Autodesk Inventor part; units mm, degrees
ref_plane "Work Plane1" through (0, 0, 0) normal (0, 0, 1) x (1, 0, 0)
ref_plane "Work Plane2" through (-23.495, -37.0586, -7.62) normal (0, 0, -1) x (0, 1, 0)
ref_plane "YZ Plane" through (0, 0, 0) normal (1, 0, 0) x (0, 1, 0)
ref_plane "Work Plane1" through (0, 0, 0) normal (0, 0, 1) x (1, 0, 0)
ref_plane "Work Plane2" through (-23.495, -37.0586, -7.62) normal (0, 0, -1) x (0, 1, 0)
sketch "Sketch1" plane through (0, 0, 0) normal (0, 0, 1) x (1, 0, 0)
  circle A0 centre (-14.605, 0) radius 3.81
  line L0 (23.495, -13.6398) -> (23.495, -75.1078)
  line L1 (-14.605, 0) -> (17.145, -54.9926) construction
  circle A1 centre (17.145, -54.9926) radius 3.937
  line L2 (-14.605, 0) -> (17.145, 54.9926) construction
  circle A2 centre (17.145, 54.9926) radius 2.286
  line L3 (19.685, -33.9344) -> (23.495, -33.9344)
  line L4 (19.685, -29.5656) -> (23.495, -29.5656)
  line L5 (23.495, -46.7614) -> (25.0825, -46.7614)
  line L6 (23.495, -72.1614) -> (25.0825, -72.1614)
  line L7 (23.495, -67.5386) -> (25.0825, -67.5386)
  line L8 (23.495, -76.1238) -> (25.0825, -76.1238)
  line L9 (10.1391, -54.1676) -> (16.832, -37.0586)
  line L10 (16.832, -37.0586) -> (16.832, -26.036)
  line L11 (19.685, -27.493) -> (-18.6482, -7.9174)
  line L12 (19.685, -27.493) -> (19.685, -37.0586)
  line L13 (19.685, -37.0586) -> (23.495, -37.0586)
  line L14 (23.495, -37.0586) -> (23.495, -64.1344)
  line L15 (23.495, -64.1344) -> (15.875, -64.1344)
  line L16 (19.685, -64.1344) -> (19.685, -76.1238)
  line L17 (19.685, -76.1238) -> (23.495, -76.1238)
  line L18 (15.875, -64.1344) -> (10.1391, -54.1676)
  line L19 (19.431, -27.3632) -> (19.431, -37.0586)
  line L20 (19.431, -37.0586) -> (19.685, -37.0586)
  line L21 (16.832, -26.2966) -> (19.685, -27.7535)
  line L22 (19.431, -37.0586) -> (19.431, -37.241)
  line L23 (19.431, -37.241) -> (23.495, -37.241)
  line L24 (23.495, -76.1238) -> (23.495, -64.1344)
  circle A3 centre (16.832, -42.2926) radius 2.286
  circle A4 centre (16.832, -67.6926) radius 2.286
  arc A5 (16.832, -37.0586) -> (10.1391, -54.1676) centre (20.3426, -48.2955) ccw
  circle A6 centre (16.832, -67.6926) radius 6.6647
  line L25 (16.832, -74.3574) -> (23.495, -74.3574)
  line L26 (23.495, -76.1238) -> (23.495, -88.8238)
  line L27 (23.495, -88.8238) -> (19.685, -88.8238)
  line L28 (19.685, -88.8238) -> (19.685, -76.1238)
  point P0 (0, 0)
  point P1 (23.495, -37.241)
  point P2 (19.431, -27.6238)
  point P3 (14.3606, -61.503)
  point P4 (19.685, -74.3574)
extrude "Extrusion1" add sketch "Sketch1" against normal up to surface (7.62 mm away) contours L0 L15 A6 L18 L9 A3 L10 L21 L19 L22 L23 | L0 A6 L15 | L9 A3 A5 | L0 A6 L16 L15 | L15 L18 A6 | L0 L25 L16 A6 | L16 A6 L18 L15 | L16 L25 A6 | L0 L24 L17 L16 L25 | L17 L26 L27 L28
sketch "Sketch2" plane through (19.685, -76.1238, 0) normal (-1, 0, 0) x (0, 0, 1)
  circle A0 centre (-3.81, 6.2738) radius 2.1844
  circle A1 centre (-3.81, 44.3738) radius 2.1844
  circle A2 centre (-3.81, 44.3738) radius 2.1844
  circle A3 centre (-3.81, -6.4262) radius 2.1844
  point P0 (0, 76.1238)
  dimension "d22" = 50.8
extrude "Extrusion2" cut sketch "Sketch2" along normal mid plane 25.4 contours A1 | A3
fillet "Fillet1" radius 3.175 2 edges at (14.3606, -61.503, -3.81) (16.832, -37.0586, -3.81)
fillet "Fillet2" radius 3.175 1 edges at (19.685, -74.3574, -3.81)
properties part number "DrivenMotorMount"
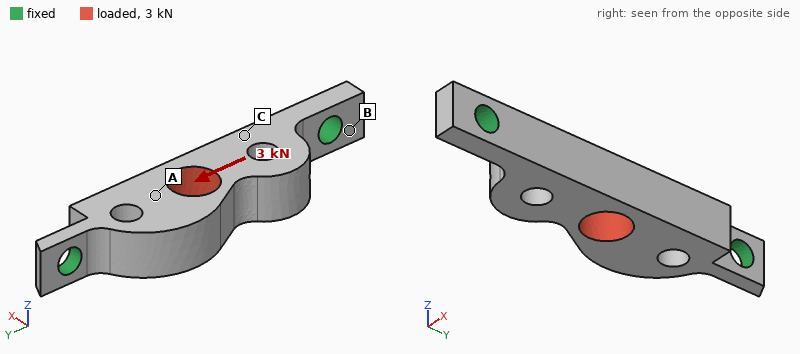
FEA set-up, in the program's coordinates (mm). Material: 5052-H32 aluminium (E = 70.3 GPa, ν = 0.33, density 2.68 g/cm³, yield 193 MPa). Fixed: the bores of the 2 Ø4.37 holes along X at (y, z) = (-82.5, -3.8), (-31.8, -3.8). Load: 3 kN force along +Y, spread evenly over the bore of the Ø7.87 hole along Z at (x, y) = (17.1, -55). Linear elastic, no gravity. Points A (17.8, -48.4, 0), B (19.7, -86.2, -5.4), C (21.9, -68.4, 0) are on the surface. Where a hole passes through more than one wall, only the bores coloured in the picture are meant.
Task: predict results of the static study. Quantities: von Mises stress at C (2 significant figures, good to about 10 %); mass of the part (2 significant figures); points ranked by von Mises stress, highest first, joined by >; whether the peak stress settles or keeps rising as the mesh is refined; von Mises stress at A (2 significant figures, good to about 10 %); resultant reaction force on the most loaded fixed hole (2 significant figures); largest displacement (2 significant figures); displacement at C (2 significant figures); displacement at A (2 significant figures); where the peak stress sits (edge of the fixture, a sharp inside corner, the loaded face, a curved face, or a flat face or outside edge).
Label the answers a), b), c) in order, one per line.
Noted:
a) 34 MPa
b) 9.3 g
c) C > A > B
d) keeps rising
e) 23 MPa
f) 1.6 kN
g) 18 µm
h) 8.3 µm
i) 13 µm
j) edge of the fixture
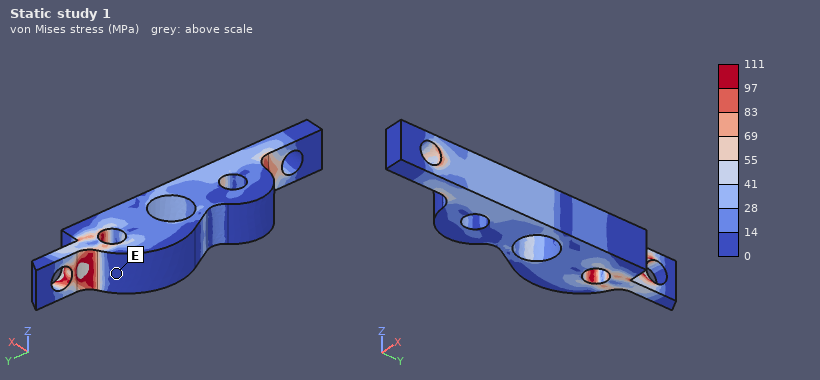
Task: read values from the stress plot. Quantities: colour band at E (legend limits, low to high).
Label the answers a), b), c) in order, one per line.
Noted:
a) 0 to 14 MPa
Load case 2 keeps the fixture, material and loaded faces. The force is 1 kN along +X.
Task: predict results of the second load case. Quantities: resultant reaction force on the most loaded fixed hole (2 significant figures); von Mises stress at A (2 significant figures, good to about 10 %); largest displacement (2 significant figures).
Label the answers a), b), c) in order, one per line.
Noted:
a) 570 N
b) 20 MPa
c) 45 µm
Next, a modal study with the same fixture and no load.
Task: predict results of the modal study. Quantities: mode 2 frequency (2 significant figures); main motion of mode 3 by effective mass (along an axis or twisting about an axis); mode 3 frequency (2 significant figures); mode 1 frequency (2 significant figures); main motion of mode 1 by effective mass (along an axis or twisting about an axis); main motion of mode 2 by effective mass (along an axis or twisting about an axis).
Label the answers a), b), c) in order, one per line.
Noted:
a) 11 kHz
b) along Z
c) 12 kHz
d) 7800 Hz
e) along Z
f) along X
